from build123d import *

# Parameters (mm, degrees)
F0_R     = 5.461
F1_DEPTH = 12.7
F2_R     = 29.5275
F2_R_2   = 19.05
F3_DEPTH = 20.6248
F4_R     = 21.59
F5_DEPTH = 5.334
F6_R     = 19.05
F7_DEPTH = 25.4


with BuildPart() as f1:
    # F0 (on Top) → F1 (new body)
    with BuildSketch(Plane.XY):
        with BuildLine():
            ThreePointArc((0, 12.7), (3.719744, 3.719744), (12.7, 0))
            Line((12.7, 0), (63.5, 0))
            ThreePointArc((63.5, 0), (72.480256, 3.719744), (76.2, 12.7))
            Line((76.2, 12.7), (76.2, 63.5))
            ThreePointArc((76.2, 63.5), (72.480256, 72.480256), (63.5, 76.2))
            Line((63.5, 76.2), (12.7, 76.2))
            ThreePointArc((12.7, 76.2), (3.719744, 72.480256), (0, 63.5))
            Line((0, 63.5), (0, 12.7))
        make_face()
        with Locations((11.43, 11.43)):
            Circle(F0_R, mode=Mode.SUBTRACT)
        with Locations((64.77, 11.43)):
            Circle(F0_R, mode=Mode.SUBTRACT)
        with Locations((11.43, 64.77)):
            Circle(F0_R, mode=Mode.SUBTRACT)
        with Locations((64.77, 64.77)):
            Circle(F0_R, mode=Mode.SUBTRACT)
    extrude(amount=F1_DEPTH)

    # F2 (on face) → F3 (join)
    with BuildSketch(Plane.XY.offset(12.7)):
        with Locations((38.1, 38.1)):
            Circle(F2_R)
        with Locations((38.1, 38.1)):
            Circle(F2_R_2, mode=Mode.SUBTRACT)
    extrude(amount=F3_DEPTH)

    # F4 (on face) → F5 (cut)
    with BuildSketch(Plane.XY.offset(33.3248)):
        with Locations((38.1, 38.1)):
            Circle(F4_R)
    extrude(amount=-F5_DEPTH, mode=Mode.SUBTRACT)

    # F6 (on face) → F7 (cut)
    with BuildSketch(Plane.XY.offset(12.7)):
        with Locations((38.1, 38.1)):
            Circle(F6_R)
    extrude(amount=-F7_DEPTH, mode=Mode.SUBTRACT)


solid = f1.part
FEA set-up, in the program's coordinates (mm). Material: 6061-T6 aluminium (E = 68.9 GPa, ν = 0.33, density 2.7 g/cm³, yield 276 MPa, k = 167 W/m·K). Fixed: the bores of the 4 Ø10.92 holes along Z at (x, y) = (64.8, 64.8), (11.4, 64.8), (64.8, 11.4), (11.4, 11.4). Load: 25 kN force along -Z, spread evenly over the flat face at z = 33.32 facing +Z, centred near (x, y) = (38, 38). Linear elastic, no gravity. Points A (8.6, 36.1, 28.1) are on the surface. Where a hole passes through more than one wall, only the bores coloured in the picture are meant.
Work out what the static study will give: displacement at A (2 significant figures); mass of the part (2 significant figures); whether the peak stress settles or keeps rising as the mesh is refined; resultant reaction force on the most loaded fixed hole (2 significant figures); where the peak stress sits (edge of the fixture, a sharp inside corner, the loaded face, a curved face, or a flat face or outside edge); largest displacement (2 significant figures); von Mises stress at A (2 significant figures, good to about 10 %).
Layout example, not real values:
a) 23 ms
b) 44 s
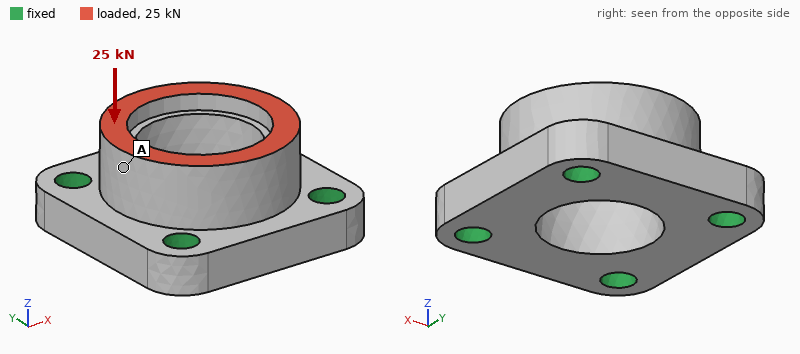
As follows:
a) 15 µm
b) 230 g
c) keeps rising
d) 6.5 kN
e) edge of the fixture
f) 17 µm
g) 19 MPa
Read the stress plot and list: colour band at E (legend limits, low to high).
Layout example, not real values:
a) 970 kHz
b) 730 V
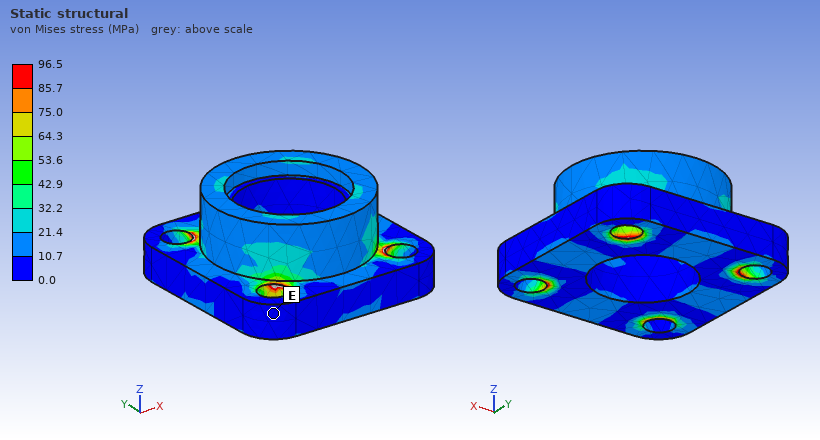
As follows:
a) 0.0 to 10.7 MPa
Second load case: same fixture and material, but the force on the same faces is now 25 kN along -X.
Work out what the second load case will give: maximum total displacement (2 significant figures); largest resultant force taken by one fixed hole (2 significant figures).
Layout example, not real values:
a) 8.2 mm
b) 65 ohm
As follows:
a) 71 µm
b) 9.1 kN
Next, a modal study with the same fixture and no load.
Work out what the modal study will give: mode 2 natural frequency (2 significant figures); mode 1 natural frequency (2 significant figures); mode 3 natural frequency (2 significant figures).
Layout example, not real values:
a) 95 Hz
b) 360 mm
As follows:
a) 17 kHz
b) 15 kHz
c) 17 kHz
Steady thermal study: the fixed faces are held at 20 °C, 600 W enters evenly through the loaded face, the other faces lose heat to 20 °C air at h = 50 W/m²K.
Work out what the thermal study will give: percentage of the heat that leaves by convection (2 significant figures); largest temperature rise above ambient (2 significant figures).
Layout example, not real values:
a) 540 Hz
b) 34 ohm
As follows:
a) 4.2 %
b) 78 K
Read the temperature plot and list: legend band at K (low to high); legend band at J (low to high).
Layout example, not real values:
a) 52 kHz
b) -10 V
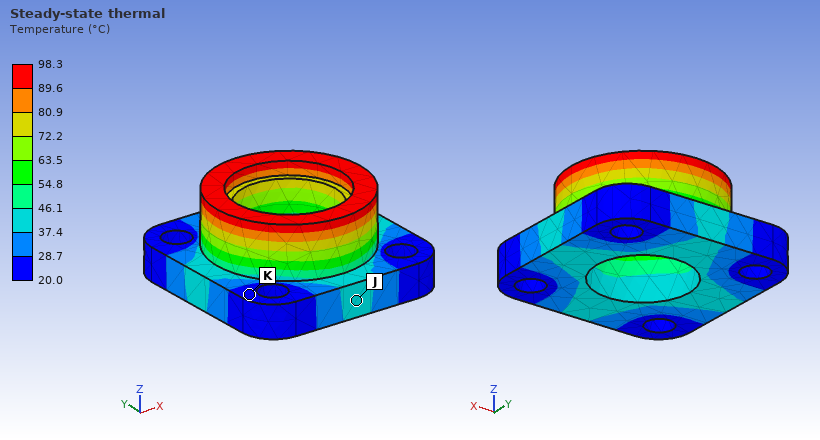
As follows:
a) 20.0 to 28.7 °C
b) 37.4 to 46.1 °C
